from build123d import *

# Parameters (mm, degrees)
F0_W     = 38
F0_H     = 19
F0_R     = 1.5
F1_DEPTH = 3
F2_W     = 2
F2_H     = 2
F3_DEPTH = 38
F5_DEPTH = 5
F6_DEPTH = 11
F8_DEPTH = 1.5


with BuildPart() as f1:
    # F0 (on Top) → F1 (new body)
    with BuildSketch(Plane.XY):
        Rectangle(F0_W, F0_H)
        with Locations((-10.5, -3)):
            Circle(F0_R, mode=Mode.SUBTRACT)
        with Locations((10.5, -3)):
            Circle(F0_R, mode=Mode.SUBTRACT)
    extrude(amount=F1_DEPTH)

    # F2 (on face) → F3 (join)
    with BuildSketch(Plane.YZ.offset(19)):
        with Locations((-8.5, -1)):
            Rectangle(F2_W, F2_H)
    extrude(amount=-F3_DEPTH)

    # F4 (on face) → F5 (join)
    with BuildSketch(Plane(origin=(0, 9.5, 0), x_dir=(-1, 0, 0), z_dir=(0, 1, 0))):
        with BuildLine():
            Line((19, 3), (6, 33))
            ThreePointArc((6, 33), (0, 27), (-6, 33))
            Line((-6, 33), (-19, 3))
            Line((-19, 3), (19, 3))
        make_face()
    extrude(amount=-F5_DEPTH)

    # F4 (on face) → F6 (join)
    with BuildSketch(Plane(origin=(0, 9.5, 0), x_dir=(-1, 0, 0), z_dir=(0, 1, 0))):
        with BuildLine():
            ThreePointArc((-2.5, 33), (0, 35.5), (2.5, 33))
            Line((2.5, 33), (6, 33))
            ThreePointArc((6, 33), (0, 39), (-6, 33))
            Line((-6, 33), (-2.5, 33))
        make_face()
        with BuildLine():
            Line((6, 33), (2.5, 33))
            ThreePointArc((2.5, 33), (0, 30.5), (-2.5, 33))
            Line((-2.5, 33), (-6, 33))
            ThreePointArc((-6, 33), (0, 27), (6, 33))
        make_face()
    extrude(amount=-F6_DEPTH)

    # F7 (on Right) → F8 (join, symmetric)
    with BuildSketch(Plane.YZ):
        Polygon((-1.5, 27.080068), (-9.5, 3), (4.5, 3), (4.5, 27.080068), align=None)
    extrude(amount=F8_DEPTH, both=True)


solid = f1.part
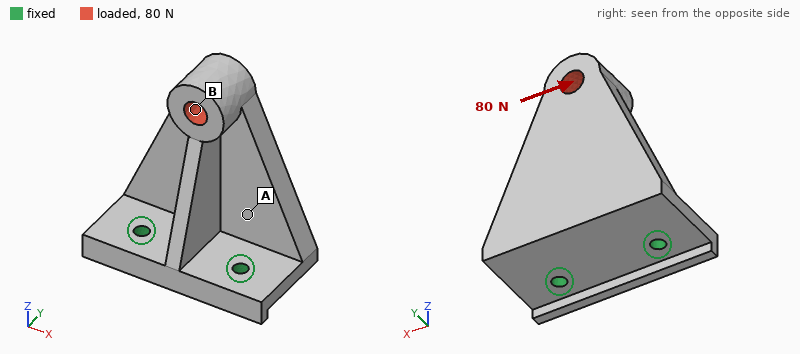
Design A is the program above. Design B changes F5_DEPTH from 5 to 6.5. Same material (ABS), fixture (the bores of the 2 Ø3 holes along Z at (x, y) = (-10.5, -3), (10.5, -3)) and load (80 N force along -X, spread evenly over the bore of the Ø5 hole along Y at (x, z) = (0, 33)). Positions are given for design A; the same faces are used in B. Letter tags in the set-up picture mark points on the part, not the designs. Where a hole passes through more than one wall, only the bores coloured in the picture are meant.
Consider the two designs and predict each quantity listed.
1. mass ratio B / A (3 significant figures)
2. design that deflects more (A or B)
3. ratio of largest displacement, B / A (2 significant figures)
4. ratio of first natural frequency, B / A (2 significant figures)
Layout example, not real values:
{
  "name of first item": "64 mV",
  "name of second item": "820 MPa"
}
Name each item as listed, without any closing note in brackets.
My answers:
{
  "mass ratio B / A": "1.12",
  "design that deflects more": "A",
  "ratio of largest displacement, B / A": "0.66",
  "ratio of first natural frequency, B / A": "0.96"
}
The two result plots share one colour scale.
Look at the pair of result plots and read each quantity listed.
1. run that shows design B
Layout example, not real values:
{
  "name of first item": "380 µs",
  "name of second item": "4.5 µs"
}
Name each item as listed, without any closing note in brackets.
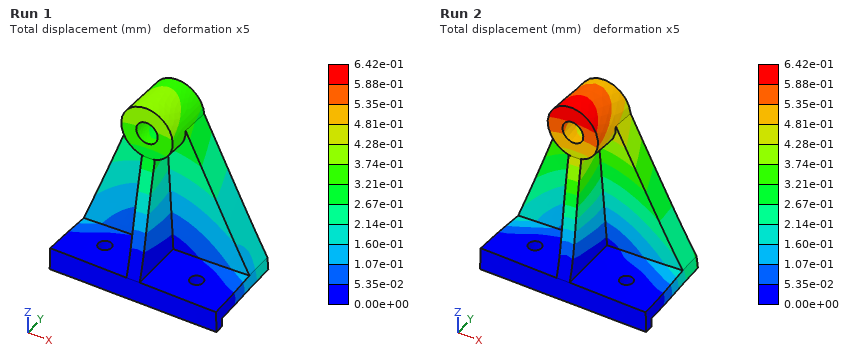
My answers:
{
  "run that shows design B": "Run 1"
}
